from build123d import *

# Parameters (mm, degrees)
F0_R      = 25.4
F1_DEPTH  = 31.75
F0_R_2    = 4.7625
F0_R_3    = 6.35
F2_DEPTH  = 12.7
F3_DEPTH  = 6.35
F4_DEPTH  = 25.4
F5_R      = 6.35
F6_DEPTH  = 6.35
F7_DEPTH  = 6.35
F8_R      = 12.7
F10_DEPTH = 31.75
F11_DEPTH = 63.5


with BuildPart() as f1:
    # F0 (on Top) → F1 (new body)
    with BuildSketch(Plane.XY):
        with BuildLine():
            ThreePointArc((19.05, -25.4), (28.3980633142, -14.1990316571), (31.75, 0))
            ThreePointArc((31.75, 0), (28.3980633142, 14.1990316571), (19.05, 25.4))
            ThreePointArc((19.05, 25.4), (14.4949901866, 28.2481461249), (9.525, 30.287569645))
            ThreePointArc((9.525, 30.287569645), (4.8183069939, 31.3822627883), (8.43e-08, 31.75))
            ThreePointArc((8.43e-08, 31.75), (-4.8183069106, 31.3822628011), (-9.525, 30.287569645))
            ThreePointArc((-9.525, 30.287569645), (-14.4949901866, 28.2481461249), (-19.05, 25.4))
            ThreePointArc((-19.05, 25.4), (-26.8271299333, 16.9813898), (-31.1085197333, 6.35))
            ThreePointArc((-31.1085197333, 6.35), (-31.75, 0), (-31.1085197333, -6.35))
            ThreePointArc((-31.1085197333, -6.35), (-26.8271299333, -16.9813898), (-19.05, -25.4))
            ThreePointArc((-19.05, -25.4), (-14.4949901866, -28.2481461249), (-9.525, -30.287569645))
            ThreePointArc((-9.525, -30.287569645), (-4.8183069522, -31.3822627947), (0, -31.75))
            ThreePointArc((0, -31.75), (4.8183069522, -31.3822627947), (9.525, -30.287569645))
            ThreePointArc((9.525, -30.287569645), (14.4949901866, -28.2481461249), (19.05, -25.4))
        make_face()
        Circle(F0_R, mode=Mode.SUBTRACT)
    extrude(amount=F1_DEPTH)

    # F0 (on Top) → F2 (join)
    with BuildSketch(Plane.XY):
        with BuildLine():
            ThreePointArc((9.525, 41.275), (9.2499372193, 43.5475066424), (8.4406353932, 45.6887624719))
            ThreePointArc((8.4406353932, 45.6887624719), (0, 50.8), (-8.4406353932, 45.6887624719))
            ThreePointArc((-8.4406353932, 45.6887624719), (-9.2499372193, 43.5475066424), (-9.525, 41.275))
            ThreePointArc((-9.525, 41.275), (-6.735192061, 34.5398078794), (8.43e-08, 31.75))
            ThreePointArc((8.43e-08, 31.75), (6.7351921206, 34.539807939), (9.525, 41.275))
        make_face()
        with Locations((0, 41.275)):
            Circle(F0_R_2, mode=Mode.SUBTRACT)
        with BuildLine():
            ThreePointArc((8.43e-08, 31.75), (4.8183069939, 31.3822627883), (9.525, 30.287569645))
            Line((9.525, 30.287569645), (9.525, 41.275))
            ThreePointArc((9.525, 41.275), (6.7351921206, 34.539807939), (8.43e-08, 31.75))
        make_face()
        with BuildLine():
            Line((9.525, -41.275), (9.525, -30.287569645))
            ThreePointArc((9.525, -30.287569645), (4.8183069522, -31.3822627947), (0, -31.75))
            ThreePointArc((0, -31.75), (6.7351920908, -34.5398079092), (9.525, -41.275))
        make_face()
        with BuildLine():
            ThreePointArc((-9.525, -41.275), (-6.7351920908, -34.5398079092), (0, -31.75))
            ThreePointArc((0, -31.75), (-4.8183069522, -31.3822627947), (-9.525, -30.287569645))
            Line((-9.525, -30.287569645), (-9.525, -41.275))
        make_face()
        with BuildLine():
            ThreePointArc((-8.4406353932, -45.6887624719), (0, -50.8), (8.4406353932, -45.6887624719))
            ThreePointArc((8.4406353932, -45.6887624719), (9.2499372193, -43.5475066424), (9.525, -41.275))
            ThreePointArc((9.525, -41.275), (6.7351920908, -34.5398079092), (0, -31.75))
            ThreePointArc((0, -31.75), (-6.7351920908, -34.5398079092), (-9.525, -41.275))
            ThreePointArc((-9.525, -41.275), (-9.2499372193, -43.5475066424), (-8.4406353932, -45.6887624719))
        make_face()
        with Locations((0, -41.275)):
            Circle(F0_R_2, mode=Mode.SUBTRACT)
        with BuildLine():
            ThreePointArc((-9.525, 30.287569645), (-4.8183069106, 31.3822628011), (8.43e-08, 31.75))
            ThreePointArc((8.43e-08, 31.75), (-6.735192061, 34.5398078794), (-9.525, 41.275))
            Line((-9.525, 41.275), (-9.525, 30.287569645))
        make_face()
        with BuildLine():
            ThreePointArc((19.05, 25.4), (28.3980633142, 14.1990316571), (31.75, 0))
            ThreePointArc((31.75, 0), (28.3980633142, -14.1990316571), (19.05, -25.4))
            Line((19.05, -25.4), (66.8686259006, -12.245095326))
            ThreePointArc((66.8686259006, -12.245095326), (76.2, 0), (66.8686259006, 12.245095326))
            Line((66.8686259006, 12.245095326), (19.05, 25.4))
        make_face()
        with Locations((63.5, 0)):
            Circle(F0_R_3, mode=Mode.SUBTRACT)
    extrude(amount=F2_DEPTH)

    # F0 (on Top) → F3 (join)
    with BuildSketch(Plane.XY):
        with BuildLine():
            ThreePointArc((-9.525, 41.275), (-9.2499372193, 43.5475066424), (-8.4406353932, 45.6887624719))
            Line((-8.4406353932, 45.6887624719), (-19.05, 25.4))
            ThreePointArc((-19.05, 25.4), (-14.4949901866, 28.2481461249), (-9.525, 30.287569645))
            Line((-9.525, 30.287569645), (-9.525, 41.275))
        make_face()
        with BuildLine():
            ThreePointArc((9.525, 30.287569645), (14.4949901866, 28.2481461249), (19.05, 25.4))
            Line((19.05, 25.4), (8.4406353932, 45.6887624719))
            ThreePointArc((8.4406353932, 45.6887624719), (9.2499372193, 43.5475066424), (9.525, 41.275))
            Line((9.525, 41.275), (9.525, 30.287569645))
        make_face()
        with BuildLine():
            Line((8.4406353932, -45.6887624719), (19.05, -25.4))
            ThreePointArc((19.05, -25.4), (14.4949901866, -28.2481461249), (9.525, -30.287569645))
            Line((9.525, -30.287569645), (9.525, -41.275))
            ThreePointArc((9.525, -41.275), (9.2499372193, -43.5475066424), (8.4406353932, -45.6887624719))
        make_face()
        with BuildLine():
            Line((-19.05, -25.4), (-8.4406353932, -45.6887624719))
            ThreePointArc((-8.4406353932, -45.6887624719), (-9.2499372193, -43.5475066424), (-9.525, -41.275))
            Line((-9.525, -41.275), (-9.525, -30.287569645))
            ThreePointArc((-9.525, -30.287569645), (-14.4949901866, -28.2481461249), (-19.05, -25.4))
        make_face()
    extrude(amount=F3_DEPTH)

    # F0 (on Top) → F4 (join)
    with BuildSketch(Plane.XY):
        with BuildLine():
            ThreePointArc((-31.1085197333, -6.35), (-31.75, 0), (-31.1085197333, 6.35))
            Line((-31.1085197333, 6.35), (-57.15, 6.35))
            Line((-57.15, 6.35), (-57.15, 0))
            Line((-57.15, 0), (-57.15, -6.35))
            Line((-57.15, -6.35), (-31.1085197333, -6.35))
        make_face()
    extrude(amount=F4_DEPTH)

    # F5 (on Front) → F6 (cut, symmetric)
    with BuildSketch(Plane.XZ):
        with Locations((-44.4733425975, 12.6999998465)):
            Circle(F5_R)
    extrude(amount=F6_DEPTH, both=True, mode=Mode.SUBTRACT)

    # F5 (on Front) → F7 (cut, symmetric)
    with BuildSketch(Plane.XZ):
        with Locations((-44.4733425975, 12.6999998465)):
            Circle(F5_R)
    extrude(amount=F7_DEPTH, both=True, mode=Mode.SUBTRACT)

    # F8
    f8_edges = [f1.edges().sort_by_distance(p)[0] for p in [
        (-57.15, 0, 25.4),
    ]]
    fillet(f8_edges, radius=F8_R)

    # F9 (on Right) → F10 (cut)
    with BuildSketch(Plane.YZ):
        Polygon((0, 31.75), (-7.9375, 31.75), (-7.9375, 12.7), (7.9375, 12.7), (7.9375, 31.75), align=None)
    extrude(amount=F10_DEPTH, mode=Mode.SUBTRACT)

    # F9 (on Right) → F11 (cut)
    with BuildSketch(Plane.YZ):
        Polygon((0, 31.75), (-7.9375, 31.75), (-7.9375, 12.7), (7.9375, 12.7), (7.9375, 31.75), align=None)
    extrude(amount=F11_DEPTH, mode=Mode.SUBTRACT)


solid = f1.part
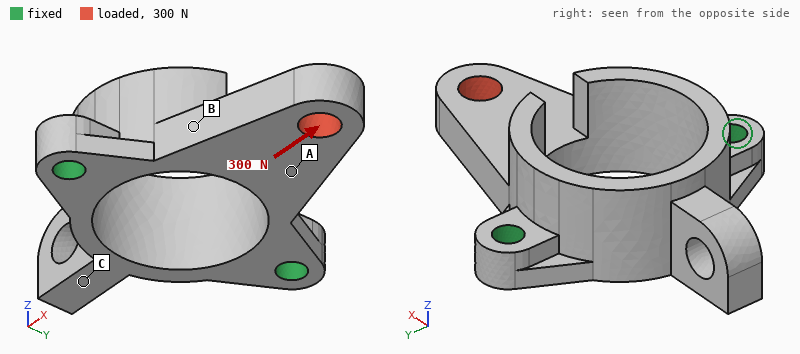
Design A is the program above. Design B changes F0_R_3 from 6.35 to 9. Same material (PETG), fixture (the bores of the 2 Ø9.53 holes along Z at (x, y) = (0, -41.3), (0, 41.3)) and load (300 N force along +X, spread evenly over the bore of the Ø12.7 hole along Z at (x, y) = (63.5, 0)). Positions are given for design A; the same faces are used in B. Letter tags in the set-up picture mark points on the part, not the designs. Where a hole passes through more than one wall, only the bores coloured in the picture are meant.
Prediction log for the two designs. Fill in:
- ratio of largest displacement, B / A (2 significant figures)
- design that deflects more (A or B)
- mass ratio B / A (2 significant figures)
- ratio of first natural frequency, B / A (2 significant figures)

1.2
B
0.98
1.1
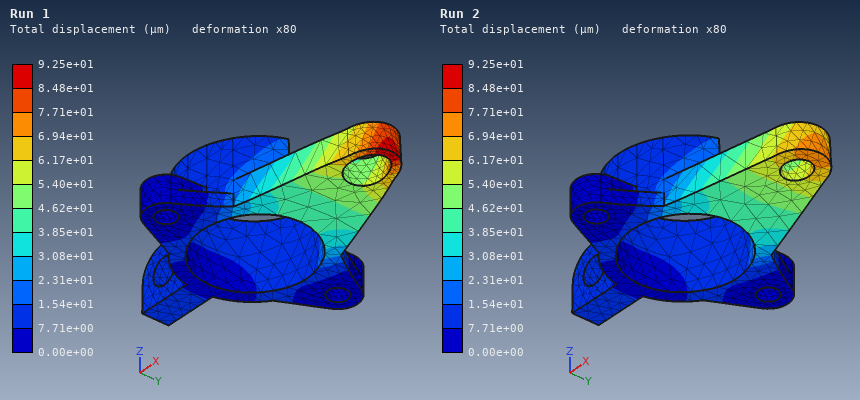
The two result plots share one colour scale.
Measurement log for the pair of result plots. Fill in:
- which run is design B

Run 1
